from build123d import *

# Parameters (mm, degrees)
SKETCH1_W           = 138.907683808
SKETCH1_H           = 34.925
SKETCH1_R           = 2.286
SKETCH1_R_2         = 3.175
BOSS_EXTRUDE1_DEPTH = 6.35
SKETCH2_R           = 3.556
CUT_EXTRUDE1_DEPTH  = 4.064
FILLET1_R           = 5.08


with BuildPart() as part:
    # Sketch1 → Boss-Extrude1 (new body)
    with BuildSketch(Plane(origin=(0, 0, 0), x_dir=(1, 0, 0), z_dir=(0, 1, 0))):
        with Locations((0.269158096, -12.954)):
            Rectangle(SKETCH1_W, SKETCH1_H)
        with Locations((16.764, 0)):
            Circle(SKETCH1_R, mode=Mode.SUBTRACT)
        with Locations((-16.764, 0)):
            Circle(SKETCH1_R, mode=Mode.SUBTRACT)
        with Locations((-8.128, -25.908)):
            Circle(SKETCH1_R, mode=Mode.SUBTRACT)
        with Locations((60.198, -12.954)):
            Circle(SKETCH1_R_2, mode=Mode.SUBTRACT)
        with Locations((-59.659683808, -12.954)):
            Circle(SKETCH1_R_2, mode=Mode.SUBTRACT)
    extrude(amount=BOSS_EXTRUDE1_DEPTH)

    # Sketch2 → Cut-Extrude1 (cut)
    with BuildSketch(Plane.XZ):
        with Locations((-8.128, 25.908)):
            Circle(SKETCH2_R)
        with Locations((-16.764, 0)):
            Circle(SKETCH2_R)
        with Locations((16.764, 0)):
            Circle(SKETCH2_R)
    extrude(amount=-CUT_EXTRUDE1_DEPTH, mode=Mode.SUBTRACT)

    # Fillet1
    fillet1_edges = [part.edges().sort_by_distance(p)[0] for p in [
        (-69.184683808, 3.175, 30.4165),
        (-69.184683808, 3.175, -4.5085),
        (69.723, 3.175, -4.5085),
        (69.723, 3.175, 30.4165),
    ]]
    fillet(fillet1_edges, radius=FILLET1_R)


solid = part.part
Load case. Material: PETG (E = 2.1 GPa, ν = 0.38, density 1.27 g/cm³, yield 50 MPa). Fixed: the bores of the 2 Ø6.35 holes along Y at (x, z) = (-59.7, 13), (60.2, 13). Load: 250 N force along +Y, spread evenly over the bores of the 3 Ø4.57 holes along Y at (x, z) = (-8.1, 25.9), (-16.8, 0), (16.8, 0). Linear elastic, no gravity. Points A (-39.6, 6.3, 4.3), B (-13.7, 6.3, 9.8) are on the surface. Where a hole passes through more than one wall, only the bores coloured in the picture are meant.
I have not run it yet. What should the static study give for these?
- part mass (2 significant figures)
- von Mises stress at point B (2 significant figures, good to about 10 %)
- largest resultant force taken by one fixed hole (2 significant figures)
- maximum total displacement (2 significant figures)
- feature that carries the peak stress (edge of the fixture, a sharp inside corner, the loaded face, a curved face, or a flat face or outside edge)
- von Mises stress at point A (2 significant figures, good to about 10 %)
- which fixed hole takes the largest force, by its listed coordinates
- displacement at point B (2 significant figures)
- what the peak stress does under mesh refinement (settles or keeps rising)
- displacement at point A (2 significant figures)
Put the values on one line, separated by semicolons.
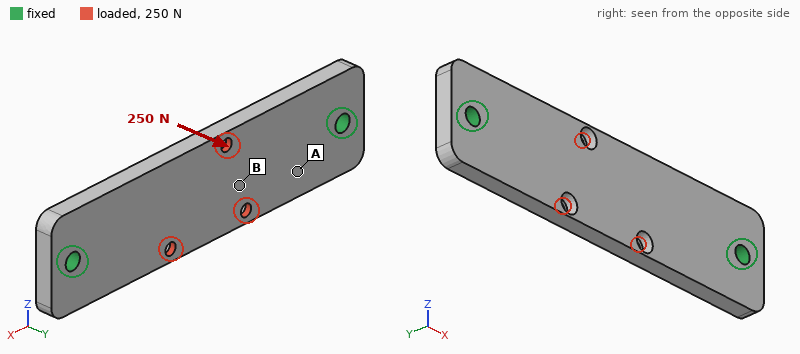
38 g; 11 MPa; 140 N; 1.6 mm; edge of the fixture; 5.0 MPa; (-59.7, 13); 1.3 mm; keeps rising; 0.47 mm
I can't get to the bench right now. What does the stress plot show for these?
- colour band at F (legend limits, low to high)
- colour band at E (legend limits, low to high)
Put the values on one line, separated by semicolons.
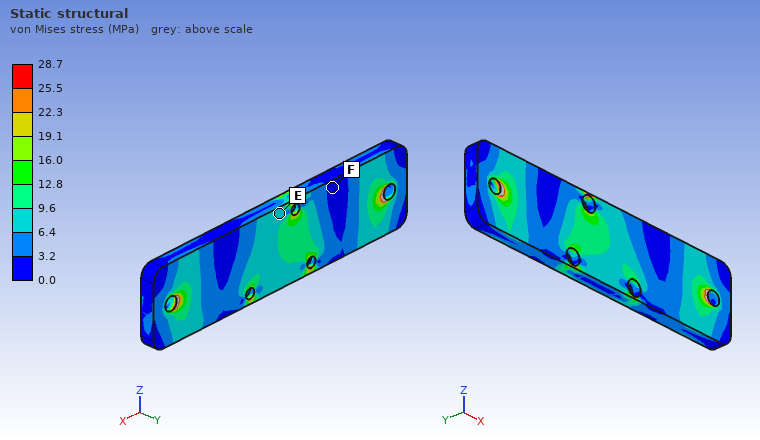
0.0 to 3.2 MPa; 6.4 to 9.6 MPa
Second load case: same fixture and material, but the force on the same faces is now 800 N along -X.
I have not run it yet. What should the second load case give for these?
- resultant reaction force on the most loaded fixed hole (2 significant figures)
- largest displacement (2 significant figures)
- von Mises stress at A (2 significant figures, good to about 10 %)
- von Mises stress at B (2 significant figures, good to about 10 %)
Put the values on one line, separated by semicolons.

420 N; 0.10 mm; 2.8 MPa; 1.3 MPa
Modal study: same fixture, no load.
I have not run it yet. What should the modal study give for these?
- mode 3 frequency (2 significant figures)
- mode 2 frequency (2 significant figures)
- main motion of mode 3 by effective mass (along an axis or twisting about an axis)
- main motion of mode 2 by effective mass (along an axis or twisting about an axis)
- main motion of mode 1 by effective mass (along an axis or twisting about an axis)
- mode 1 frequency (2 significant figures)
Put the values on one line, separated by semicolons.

1400 Hz; 1100 Hz; along Z; twisting about X; along Y; 570 Hz
